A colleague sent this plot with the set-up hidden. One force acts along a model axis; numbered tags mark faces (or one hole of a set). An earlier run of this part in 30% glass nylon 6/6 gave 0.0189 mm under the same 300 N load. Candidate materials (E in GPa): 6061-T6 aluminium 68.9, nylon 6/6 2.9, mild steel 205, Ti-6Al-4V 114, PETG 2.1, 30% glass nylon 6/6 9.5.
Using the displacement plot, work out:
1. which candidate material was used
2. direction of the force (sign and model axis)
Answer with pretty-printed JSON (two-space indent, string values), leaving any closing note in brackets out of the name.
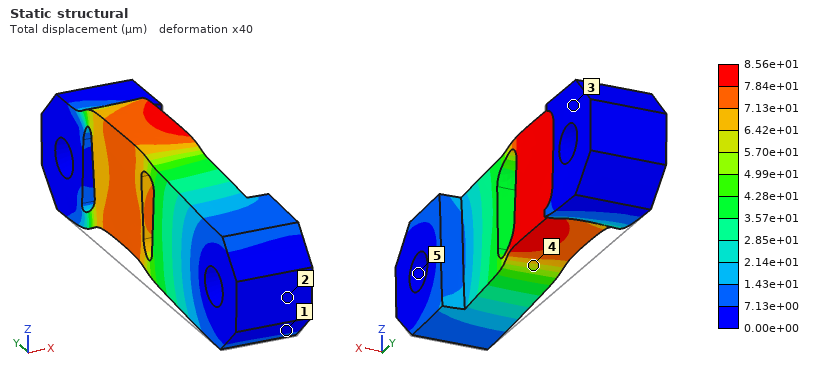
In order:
{
  "which candidate material was used": "PETG",
  "direction of the force": "+Z"
}
